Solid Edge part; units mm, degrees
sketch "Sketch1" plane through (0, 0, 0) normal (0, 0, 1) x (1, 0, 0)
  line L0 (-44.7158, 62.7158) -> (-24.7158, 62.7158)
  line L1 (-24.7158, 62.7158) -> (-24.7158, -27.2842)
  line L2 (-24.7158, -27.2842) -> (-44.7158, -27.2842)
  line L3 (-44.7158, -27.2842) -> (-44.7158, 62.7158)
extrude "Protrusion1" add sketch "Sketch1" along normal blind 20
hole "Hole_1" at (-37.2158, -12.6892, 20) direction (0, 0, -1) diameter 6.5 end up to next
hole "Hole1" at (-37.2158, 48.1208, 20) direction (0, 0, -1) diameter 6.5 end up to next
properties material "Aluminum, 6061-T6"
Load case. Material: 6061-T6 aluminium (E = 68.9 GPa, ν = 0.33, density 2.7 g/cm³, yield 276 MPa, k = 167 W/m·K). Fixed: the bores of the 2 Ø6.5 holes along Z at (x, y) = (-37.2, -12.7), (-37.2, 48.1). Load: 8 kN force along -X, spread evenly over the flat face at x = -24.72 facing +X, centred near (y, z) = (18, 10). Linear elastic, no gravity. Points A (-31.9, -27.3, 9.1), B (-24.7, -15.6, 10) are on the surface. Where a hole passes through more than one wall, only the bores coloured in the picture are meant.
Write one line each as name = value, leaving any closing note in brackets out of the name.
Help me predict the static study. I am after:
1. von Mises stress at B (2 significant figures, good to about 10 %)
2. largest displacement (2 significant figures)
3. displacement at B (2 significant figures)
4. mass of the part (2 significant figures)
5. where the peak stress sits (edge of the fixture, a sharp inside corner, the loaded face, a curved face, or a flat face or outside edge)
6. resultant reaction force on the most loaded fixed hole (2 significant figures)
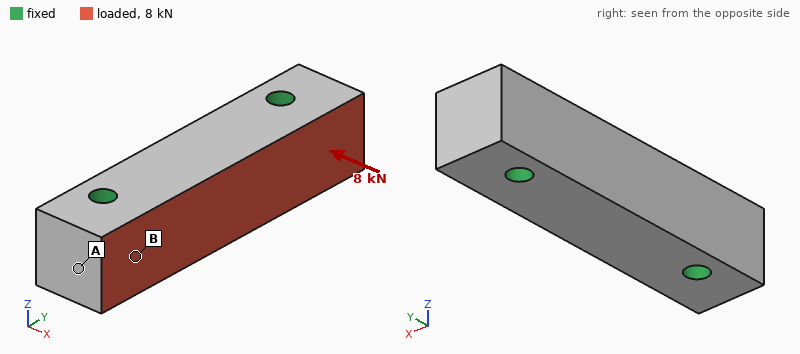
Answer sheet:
von Mises stress at B = 11 MPa
largest displacement = 9.5 µm
displacement at B = 1.6 µm
mass of the part = 94 g
where the peak stress sits = edge of the fixture
resultant reaction force on the most loaded fixed hole = 4.1 kN
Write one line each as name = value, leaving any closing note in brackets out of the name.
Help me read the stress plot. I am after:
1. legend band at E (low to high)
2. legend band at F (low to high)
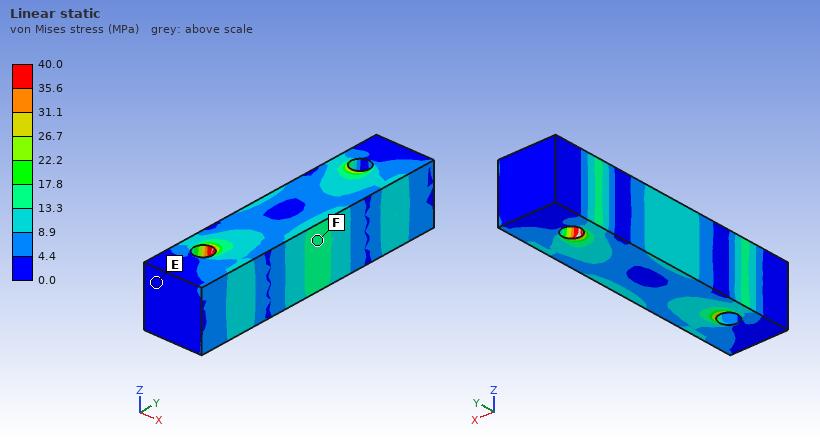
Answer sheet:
legend band at E = 0.0 to 4.4 MPa
legend band at F = 13.3 to 17.8 MPa
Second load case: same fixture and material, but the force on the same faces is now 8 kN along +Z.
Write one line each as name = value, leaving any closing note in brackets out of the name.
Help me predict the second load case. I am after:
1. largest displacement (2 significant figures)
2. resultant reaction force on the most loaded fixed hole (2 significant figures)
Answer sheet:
largest displacement = 20 µm
resultant reaction force on the most loaded fixed hole = 4.0 kN
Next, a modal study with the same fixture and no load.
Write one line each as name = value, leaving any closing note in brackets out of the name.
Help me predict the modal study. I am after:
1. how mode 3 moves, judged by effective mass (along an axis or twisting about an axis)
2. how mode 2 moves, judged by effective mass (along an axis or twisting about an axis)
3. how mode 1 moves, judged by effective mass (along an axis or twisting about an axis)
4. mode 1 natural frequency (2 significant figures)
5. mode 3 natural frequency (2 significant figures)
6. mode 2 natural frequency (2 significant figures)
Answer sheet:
how mode 3 moves, judged by effective mass = twisting about Y
how mode 2 moves, judged by effective mass = along Z
how mode 1 moves, judged by effective mass = along X
mode 1 natural frequency = 16 kHz
mode 3 natural frequency = 24 kHz
mode 2 natural frequency = 18 kHz
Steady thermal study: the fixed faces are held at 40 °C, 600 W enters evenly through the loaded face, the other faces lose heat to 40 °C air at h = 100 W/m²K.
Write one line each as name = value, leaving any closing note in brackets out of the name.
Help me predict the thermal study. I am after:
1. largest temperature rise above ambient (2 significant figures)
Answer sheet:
largest temperature rise above ambient = 61 K
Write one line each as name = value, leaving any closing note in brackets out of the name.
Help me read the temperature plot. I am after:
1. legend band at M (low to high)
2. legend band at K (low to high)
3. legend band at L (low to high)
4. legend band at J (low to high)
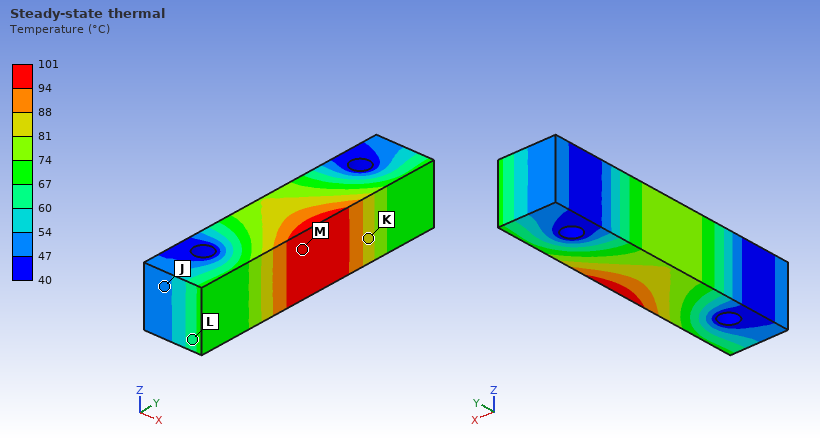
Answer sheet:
legend band at M = 94 to 101 °C
legend band at K = 81 to 88 °C
legend band at L = 60 to 67 °C
legend band at J = 47 to 54 °C
